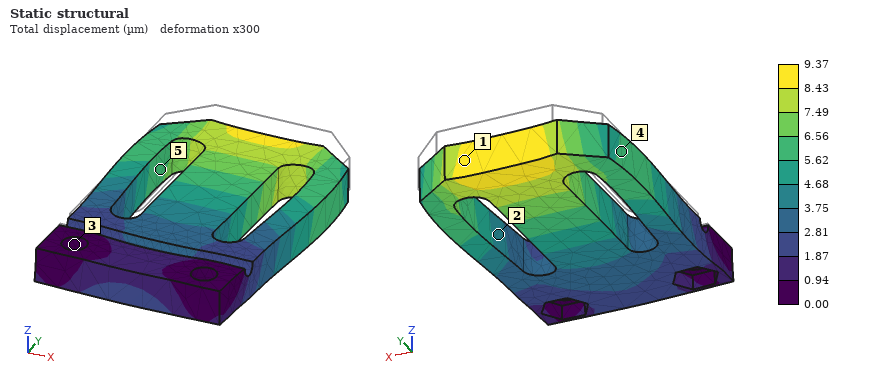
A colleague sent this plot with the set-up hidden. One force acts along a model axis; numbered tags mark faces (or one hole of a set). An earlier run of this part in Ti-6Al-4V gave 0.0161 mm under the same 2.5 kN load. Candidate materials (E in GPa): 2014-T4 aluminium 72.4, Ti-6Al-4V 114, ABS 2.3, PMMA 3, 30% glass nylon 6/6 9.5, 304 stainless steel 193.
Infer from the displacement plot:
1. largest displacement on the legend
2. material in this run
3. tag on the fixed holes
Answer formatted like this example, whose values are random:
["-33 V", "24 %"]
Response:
["9.37 µm", "304 stainless steel", "3"]
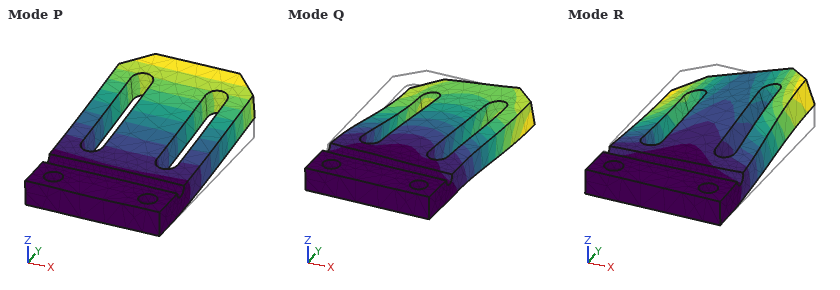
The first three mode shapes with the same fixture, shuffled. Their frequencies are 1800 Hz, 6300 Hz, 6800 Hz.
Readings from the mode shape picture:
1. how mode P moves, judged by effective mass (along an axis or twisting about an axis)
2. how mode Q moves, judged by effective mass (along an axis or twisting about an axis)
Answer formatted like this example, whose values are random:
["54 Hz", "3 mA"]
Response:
["along Z", "along X"]
